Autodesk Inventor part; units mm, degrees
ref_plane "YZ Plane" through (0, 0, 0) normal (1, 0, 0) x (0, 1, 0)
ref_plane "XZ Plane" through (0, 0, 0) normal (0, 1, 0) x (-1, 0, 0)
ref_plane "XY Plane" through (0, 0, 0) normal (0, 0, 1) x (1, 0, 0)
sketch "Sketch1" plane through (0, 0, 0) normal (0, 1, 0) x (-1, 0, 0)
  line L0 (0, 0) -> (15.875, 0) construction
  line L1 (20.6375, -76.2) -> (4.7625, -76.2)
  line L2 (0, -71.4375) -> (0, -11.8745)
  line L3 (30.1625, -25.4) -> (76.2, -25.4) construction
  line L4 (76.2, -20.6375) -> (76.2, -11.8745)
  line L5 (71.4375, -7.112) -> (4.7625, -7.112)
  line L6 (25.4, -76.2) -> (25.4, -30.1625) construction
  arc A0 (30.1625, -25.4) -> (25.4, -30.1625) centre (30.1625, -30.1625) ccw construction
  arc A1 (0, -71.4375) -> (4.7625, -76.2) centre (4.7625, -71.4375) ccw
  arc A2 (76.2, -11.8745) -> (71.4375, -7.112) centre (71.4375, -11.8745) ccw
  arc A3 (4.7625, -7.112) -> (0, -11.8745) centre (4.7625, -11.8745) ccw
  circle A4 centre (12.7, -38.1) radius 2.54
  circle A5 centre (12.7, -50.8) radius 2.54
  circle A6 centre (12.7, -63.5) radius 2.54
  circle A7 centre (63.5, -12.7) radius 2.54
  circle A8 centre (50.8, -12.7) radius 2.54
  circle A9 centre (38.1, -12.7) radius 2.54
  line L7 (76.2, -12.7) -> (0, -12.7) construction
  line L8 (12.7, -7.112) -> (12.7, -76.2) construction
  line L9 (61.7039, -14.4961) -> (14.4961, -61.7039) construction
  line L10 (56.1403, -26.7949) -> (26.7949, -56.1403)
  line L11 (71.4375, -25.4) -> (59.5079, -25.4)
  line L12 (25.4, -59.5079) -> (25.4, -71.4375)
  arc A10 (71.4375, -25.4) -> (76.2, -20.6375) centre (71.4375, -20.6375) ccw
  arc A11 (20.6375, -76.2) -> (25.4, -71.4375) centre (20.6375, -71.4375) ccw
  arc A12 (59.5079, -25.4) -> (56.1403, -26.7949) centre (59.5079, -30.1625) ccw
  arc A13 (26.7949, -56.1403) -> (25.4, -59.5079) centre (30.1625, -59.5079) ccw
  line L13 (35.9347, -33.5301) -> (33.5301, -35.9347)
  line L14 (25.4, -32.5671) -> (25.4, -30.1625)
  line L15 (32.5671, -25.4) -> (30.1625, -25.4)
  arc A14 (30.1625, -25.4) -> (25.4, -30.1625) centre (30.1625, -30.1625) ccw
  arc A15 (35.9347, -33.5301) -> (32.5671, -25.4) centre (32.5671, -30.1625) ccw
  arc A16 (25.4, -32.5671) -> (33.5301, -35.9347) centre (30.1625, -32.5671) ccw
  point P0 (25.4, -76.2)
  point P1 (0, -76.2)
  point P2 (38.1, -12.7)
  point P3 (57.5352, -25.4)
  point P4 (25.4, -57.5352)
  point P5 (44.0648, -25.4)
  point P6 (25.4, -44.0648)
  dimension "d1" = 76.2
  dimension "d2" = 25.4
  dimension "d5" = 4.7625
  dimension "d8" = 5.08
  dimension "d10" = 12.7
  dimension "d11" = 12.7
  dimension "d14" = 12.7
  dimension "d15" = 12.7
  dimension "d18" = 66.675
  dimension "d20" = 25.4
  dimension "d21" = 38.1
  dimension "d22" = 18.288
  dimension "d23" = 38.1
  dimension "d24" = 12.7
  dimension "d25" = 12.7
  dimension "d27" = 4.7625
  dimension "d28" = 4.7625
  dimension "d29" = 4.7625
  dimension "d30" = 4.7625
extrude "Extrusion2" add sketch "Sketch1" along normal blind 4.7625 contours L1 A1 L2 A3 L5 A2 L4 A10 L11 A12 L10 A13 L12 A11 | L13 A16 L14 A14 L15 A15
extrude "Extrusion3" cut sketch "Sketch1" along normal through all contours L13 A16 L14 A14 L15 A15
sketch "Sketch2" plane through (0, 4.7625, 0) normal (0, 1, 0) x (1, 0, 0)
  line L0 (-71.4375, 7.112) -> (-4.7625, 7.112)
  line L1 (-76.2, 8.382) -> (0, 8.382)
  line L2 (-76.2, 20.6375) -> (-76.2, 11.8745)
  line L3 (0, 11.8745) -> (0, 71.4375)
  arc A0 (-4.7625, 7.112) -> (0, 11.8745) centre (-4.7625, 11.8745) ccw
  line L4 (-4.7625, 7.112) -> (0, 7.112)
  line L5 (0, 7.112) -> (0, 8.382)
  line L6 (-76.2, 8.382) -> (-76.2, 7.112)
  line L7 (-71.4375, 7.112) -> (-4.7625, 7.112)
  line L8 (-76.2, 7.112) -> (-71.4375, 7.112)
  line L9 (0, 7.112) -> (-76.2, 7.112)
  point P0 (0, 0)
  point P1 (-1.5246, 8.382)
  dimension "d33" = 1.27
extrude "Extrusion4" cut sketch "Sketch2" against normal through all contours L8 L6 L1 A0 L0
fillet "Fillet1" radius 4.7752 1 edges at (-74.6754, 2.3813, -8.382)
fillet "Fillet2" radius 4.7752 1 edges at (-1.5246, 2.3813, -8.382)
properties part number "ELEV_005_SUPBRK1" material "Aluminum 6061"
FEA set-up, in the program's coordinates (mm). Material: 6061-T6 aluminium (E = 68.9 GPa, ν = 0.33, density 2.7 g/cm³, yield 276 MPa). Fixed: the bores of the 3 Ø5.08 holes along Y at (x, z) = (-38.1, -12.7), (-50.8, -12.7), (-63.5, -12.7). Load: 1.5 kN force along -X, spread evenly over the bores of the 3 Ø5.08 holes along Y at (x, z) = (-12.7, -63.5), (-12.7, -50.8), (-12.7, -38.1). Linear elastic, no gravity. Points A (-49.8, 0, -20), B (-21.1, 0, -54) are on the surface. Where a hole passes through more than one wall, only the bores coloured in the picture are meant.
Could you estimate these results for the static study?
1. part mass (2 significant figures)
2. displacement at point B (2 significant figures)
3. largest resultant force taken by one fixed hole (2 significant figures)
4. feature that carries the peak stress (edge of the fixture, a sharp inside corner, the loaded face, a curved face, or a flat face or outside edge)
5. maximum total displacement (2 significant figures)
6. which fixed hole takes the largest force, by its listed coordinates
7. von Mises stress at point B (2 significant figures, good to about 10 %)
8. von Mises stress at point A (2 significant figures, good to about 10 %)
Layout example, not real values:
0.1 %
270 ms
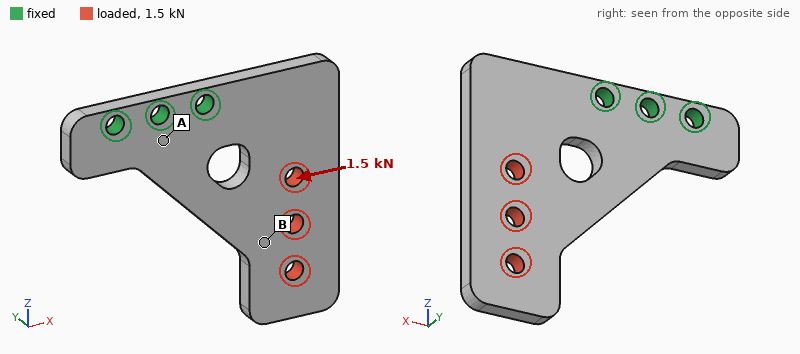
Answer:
37 g
0.087 mm
2.3 kN
edge of the fixture
0.14 mm
(-38.1, -12.7)
17 MPa
35 MPa
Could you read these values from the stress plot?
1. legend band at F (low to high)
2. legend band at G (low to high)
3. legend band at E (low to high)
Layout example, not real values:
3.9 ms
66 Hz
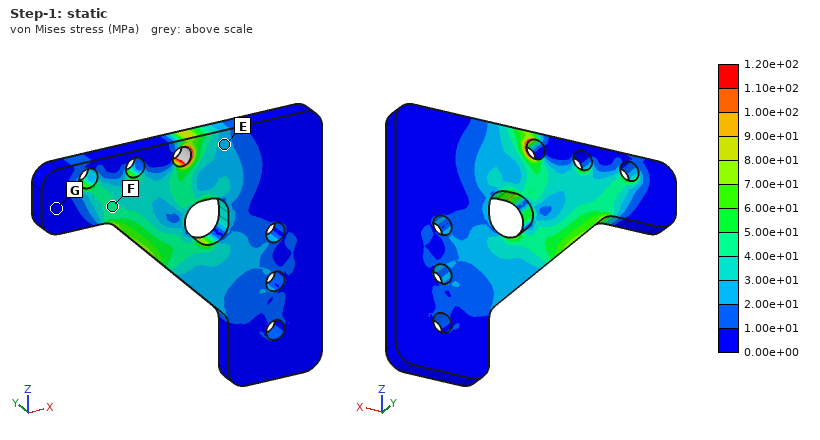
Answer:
4.00e+01 to 5.00e+01 MPa
0.00e+00 to 1.00e+01 MPa
2.00e+01 to 3.00e+01 MPa
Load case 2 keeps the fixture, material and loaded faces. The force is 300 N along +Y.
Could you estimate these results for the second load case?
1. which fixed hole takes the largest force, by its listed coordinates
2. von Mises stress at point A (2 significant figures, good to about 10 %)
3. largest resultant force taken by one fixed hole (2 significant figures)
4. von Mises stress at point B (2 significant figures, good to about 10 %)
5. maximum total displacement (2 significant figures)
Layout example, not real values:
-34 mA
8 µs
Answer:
(-38.1, -12.7)
49 MPa
530 N
18 MPa
0.97 mm
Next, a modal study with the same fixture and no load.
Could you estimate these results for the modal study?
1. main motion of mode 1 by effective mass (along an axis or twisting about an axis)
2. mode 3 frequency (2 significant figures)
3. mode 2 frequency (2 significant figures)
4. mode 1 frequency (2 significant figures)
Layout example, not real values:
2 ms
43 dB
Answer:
along Y
3900 Hz
2500 Hz
860 Hz
